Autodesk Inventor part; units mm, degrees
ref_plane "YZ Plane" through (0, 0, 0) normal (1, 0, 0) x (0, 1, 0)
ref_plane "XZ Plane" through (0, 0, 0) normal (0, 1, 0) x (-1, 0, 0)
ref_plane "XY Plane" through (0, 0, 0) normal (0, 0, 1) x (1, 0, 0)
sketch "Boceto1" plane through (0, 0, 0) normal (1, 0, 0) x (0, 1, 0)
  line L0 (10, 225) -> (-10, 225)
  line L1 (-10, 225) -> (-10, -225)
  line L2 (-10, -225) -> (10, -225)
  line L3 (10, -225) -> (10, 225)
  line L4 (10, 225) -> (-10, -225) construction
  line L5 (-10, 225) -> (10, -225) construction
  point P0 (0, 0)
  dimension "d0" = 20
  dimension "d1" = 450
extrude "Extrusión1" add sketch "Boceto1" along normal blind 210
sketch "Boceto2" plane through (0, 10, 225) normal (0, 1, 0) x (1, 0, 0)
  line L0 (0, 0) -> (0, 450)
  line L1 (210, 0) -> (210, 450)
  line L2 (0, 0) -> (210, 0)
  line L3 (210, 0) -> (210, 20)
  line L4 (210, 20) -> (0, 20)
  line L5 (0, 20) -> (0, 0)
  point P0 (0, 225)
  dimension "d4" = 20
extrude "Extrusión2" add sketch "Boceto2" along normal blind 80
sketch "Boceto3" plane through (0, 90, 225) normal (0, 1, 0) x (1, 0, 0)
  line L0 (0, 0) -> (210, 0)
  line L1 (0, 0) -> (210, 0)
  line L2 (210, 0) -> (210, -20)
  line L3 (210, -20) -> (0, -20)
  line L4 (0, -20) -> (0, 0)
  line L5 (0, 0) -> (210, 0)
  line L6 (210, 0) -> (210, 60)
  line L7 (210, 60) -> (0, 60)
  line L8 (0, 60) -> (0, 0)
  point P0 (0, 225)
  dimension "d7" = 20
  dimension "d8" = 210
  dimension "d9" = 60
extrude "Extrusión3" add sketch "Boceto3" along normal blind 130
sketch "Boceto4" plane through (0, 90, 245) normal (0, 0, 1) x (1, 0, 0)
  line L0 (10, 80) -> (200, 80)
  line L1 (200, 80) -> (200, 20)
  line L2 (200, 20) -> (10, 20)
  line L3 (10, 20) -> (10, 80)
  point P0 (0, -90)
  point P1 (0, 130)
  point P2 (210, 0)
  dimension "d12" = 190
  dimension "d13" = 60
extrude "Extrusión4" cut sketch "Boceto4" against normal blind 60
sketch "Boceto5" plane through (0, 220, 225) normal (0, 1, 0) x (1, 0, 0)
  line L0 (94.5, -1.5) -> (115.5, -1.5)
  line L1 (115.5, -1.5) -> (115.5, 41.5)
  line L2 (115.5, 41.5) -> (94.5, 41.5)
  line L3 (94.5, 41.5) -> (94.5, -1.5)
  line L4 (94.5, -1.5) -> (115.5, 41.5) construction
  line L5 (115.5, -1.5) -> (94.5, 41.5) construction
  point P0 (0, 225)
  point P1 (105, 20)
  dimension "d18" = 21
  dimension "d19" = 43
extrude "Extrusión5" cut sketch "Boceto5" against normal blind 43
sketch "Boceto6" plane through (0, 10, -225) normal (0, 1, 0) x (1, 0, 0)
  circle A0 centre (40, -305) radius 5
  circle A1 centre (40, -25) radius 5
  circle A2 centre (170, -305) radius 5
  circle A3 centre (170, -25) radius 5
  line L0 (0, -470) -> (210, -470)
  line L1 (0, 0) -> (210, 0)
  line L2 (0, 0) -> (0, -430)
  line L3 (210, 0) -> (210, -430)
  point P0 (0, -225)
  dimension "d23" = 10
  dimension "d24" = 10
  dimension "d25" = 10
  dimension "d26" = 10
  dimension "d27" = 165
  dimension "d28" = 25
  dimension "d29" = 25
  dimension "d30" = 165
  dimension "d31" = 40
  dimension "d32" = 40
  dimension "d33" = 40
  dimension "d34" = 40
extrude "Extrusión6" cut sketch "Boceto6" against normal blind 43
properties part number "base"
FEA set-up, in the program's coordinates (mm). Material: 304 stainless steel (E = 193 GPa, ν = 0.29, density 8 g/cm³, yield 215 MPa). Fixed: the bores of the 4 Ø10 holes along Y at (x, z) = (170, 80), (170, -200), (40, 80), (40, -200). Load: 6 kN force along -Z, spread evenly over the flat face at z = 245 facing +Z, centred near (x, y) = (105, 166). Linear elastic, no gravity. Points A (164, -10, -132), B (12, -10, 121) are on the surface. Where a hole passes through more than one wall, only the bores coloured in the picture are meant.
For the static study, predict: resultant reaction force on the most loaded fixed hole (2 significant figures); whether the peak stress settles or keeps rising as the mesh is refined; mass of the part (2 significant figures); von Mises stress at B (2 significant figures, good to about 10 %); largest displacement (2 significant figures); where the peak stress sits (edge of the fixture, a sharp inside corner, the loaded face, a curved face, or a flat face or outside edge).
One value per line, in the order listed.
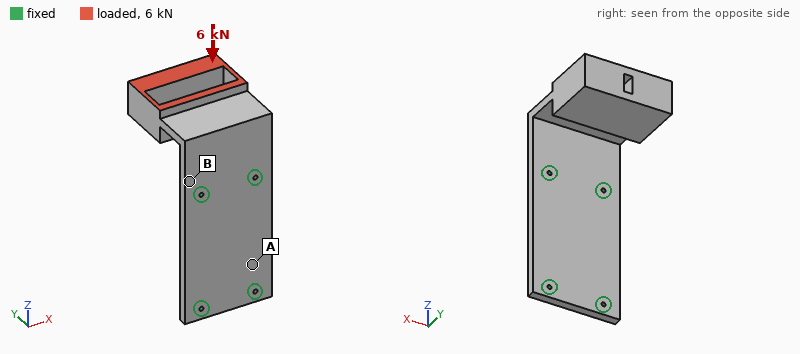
2.7 kN
keeps rising
29 kg
72 MPa
1.6 mm
edge of the fixture
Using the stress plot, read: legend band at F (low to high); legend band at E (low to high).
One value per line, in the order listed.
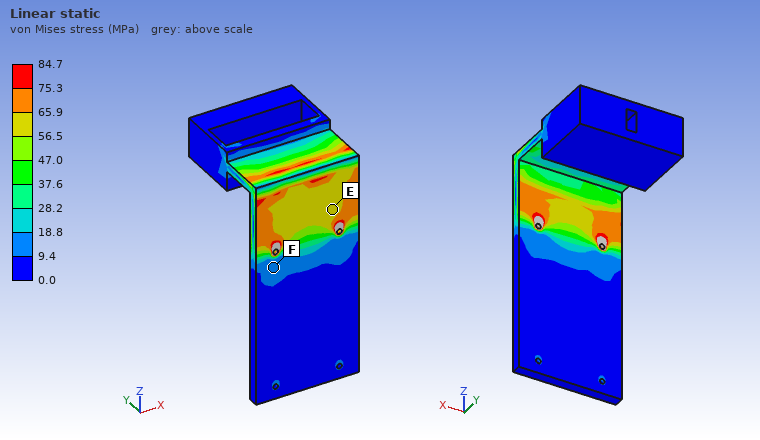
9.4 to 18.8 MPa
56.5 to 65.9 MPa
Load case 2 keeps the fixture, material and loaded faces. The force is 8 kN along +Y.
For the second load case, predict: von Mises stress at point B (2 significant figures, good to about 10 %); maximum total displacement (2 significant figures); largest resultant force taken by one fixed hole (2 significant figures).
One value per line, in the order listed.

73 MPa
1.2 mm
4.6 kN
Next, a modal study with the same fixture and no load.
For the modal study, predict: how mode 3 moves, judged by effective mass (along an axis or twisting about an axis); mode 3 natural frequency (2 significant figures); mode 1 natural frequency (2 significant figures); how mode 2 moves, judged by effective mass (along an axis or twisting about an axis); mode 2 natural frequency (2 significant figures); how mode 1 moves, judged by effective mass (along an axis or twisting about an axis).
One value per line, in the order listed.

along Y
320 Hz
100 Hz
along X
180 Hz
along Z
